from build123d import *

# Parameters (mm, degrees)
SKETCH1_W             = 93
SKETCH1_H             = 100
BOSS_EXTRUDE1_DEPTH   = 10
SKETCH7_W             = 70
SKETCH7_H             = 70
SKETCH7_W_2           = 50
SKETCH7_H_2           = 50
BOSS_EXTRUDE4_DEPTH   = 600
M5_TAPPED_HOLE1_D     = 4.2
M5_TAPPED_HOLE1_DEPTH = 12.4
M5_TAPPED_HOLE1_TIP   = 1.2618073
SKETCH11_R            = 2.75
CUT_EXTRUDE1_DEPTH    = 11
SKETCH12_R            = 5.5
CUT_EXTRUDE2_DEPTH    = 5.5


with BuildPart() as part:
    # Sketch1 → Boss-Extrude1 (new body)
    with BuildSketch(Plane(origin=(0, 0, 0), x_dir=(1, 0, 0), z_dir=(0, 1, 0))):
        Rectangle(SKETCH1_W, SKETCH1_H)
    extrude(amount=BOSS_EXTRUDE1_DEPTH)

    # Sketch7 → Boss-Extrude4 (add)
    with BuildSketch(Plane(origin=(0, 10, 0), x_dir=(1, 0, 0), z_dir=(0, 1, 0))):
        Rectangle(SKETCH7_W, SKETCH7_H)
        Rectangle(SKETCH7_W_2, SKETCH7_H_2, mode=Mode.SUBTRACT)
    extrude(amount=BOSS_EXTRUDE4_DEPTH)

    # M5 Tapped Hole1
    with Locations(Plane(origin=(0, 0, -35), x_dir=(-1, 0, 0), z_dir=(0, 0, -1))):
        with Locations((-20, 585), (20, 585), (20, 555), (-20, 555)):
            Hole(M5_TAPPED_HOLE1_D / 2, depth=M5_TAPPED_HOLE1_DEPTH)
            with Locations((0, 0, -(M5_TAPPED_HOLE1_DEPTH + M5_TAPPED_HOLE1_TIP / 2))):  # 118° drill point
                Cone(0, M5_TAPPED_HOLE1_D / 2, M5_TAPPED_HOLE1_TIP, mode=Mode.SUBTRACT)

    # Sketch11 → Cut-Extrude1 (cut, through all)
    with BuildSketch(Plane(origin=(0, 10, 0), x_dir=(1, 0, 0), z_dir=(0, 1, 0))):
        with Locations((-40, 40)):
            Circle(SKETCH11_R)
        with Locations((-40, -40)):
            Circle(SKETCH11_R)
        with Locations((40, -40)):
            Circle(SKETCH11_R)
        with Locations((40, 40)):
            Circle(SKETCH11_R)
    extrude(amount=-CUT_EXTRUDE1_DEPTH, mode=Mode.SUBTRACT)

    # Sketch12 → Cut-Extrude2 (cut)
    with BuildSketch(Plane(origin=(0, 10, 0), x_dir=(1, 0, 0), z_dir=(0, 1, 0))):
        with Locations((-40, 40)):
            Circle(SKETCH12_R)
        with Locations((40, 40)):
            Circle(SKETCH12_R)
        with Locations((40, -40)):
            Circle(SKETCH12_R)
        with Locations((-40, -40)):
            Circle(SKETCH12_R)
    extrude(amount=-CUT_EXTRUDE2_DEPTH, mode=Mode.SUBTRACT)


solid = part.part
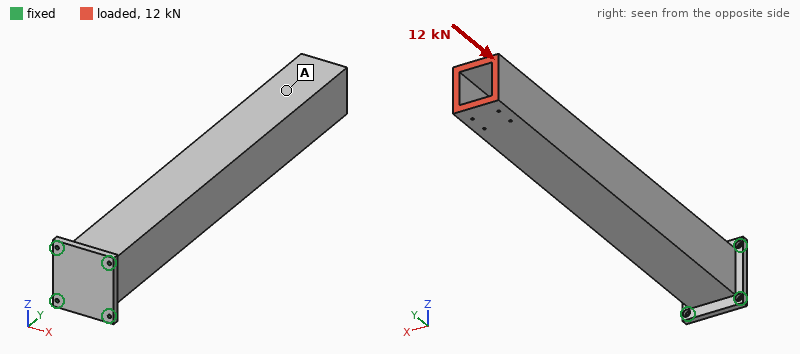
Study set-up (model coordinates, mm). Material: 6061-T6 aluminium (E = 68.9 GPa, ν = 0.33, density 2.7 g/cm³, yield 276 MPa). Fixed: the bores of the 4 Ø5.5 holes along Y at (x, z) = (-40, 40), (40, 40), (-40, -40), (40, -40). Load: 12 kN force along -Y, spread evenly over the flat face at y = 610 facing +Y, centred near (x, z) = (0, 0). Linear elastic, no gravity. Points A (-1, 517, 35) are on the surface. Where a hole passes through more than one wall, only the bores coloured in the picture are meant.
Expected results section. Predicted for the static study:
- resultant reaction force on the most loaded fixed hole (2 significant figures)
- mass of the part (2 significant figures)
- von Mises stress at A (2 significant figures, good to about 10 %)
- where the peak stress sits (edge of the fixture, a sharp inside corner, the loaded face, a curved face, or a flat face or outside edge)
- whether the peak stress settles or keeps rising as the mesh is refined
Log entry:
3.7 kN
4.1 kg
5.0 MPa
edge of the fixture
keeps rising
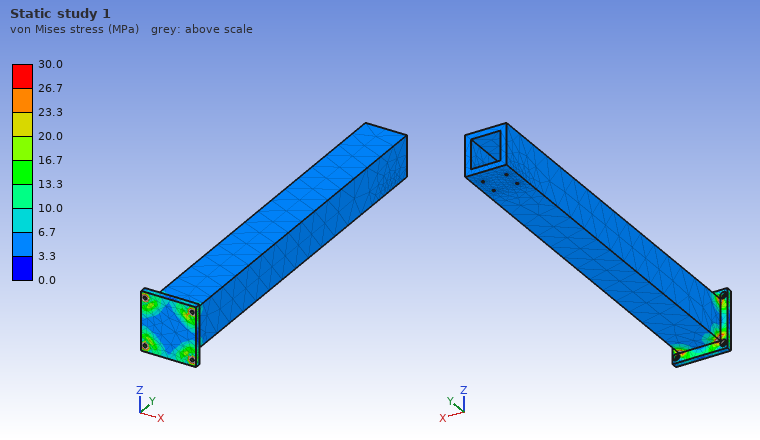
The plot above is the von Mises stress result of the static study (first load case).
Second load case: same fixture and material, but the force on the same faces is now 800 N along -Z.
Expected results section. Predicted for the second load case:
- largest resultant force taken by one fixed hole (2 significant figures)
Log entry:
3.5 kN
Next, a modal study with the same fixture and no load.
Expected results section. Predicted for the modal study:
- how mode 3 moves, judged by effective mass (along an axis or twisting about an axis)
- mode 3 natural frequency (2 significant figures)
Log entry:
along X
890 Hz
